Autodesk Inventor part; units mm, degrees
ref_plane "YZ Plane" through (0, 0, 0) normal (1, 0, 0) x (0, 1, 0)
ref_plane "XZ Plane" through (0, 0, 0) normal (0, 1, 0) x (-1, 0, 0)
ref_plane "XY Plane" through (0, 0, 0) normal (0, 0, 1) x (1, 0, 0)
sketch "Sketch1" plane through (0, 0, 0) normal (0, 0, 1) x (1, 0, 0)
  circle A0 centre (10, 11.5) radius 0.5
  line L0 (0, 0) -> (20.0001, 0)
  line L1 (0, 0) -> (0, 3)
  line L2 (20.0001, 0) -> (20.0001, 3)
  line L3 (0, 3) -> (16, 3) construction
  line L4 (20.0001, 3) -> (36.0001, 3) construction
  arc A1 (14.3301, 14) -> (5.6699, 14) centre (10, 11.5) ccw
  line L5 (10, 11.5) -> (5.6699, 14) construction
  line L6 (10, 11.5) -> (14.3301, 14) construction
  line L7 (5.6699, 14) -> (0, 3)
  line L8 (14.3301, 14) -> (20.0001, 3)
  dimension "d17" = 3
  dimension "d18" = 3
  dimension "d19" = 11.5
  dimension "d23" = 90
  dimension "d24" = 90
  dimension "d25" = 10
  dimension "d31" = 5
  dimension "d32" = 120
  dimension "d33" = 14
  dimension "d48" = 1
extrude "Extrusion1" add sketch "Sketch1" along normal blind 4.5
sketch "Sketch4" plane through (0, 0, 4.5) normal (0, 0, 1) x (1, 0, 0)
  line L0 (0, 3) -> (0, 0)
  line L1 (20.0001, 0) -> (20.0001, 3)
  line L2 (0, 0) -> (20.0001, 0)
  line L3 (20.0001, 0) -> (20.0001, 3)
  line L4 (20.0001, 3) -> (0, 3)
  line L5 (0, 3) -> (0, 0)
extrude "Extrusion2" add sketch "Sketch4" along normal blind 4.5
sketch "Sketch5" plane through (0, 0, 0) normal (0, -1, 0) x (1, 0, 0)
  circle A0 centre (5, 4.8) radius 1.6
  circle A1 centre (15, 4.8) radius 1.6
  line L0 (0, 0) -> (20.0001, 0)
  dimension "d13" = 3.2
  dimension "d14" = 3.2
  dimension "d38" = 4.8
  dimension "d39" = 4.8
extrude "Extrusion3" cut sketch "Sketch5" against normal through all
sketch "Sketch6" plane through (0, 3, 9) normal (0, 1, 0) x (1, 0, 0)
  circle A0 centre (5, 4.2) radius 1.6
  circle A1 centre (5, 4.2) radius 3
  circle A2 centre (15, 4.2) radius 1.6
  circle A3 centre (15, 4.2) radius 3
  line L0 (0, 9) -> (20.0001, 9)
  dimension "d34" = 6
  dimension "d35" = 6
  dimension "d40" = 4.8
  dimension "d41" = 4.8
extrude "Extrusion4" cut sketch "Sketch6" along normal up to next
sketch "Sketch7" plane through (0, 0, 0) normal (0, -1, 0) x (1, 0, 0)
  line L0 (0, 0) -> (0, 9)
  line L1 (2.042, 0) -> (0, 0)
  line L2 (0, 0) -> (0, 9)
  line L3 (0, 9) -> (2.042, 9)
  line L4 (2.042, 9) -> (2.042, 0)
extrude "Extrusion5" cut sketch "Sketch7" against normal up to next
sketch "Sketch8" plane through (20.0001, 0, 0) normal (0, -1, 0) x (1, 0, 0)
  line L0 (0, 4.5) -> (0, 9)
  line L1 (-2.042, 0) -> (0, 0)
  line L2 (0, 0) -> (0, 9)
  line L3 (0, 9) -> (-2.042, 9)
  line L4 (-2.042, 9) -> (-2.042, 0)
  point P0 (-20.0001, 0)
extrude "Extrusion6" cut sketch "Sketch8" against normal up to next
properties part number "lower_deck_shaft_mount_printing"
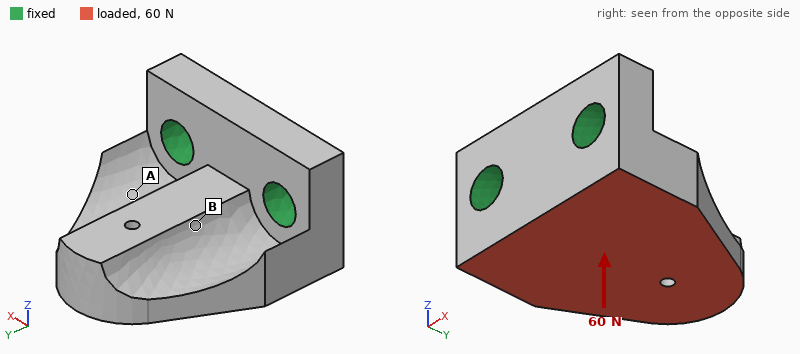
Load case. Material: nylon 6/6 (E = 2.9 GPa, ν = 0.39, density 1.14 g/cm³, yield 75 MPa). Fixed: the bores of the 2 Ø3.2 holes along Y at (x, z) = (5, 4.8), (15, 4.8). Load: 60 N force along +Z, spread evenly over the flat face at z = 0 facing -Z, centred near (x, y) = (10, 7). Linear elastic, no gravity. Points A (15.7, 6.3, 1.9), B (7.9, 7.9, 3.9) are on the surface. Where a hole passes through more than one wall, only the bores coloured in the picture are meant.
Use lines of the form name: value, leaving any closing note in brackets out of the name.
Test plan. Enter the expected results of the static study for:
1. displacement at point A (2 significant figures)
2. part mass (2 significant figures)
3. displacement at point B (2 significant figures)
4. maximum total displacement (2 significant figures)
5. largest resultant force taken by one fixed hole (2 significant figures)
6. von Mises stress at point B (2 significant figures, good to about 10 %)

displacement at point A: 0.039 mm
part mass: 1.0 g
displacement at point B: 0.060 mm
maximum total displacement: 0.17 mm
largest resultant force taken by one fixed hole: 31 N
von Mises stress at point B: 3.8 MPa
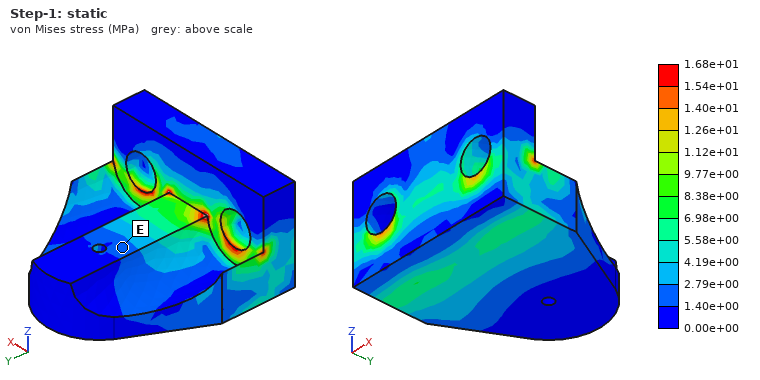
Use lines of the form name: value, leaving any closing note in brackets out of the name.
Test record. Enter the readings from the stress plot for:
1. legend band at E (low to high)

legend band at E: 1.40e+00 to 2.79e+00 MPa
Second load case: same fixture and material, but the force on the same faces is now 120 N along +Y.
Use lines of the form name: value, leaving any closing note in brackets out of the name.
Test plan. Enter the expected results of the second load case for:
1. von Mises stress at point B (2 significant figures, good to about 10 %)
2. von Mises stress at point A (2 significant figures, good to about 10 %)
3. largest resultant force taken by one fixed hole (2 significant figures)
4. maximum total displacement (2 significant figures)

von Mises stress at point B: 2.1 MPa
von Mises stress at point A: 2.0 MPa
largest resultant force taken by one fixed hole: 60 N
maximum total displacement: 0.17 mm
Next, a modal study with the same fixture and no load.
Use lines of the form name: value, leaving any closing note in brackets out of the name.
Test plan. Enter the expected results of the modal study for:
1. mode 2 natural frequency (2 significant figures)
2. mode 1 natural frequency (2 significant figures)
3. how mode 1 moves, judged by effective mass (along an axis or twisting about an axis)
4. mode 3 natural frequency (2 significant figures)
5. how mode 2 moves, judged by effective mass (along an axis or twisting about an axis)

mode 2 natural frequency: 9100 Hz
mode 1 natural frequency: 4300 Hz
how mode 1 moves, judged by effective mass: along Z
mode 3 natural frequency: 13 kHz
how mode 2 moves, judged by effective mass: along X
